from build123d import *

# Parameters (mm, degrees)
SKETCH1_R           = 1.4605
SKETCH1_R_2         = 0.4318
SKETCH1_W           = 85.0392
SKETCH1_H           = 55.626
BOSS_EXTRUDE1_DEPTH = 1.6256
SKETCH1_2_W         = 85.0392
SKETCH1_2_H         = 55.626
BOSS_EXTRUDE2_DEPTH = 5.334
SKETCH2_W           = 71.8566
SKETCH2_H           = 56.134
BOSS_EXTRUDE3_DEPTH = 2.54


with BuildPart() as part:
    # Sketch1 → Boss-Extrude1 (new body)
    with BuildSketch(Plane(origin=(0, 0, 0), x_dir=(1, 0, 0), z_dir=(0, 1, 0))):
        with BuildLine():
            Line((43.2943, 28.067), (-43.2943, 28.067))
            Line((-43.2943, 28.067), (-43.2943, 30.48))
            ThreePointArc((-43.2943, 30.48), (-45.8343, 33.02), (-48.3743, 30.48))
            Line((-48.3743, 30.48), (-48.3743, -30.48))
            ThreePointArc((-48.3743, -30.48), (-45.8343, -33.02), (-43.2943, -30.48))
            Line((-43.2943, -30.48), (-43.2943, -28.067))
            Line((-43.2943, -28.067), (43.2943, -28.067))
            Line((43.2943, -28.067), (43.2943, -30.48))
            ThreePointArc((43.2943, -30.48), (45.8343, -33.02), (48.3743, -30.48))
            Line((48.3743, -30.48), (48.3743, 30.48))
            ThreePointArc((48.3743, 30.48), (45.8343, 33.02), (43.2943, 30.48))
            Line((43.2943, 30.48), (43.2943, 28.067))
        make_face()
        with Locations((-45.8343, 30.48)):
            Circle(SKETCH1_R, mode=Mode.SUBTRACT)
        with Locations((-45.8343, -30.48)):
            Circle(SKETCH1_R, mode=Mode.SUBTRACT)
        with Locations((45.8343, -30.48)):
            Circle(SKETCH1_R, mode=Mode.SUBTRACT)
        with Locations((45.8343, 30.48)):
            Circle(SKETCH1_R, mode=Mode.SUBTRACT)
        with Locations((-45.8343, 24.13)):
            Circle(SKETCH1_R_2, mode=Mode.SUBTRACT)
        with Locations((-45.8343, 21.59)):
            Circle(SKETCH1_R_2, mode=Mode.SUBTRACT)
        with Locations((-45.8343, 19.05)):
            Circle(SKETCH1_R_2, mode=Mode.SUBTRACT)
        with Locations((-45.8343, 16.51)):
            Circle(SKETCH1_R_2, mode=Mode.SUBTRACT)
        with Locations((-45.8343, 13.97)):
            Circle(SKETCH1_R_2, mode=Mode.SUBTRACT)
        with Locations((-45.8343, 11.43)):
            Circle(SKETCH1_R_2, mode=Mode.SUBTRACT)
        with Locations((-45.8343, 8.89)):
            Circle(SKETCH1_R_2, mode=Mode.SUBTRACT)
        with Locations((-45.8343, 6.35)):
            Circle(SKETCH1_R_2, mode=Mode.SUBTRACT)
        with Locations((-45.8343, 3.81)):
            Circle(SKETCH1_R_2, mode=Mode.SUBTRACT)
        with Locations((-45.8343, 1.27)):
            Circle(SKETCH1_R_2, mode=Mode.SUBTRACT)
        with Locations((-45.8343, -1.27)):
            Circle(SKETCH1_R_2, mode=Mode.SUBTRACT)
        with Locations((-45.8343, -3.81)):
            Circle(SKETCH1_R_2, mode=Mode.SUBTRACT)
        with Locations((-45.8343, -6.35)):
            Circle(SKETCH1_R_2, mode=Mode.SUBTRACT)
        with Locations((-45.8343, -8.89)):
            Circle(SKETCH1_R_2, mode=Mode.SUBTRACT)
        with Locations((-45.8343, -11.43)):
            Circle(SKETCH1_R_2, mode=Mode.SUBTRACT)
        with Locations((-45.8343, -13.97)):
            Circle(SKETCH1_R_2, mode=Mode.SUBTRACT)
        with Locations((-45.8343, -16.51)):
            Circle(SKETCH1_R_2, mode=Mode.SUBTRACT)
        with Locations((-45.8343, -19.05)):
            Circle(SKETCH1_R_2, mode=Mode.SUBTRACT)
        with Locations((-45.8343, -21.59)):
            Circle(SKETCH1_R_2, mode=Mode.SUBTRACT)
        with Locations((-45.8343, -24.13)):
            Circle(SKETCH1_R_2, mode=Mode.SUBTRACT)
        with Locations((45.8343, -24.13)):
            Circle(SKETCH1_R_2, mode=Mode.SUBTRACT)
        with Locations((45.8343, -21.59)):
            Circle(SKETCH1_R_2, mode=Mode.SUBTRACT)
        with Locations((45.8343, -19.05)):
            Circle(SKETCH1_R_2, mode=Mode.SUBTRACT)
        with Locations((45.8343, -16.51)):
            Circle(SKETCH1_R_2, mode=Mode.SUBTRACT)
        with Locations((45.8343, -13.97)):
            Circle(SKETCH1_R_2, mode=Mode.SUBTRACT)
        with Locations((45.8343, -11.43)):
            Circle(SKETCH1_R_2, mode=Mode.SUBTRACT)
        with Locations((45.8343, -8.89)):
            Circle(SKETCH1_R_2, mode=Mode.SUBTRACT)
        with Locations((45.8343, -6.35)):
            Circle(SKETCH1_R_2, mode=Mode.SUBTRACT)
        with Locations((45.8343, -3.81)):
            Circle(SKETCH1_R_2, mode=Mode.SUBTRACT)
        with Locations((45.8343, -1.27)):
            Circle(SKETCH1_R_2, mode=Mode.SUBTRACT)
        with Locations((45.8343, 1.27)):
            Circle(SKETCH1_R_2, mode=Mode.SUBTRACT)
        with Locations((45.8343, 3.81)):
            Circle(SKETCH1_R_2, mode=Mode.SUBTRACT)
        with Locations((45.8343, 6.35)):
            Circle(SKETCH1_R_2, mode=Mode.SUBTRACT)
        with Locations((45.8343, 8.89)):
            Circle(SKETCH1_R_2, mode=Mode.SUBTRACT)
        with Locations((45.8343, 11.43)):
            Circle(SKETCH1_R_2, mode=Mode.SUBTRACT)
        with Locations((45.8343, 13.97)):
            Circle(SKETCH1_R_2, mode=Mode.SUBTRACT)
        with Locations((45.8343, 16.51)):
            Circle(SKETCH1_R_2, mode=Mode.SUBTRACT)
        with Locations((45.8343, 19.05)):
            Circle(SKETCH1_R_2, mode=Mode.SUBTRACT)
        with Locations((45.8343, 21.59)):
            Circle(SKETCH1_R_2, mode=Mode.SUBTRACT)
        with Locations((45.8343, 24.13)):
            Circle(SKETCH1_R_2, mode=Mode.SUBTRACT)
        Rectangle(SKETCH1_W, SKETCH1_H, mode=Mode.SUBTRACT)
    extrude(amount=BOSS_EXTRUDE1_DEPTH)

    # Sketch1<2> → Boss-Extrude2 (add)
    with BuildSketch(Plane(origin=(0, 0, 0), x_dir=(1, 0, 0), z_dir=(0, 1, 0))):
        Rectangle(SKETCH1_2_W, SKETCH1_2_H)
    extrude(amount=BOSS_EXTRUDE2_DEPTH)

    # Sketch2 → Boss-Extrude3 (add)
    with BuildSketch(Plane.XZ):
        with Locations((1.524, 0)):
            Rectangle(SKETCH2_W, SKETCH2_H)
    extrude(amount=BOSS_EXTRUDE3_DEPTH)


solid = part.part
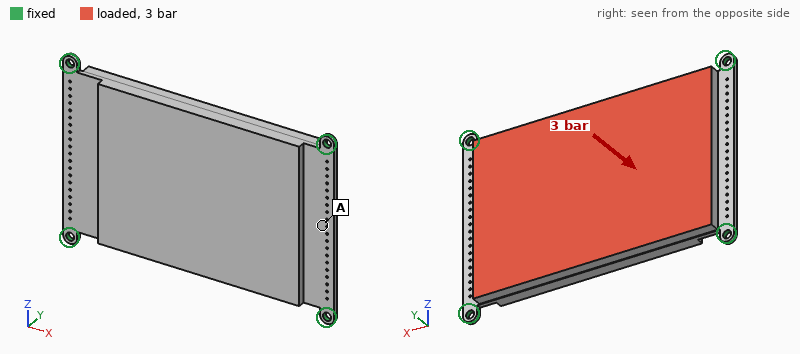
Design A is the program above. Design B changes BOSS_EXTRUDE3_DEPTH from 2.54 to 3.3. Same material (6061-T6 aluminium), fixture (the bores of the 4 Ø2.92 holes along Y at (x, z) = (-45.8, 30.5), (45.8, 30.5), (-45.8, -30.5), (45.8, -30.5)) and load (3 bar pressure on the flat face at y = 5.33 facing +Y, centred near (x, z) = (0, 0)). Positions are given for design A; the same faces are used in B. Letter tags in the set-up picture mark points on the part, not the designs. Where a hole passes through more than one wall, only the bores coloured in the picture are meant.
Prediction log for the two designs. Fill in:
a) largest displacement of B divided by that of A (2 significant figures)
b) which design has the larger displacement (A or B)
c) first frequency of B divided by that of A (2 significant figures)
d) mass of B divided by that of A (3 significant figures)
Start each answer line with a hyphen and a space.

- 0.87
- A
- 1.0
- 1.08
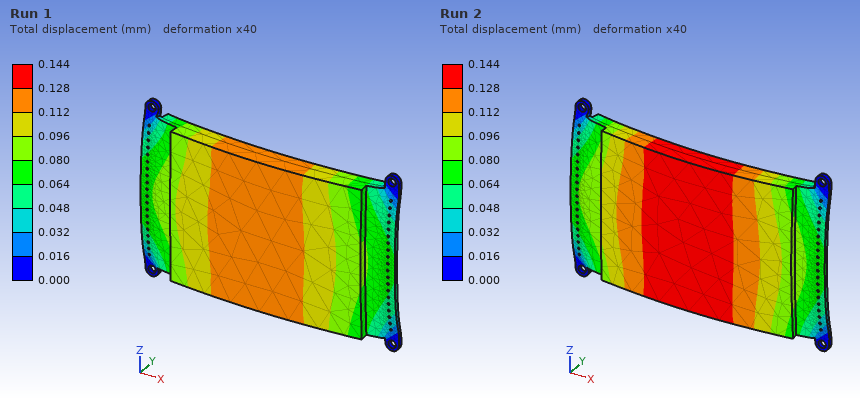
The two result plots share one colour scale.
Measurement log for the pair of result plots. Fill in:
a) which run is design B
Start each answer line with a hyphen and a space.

- Run 1
